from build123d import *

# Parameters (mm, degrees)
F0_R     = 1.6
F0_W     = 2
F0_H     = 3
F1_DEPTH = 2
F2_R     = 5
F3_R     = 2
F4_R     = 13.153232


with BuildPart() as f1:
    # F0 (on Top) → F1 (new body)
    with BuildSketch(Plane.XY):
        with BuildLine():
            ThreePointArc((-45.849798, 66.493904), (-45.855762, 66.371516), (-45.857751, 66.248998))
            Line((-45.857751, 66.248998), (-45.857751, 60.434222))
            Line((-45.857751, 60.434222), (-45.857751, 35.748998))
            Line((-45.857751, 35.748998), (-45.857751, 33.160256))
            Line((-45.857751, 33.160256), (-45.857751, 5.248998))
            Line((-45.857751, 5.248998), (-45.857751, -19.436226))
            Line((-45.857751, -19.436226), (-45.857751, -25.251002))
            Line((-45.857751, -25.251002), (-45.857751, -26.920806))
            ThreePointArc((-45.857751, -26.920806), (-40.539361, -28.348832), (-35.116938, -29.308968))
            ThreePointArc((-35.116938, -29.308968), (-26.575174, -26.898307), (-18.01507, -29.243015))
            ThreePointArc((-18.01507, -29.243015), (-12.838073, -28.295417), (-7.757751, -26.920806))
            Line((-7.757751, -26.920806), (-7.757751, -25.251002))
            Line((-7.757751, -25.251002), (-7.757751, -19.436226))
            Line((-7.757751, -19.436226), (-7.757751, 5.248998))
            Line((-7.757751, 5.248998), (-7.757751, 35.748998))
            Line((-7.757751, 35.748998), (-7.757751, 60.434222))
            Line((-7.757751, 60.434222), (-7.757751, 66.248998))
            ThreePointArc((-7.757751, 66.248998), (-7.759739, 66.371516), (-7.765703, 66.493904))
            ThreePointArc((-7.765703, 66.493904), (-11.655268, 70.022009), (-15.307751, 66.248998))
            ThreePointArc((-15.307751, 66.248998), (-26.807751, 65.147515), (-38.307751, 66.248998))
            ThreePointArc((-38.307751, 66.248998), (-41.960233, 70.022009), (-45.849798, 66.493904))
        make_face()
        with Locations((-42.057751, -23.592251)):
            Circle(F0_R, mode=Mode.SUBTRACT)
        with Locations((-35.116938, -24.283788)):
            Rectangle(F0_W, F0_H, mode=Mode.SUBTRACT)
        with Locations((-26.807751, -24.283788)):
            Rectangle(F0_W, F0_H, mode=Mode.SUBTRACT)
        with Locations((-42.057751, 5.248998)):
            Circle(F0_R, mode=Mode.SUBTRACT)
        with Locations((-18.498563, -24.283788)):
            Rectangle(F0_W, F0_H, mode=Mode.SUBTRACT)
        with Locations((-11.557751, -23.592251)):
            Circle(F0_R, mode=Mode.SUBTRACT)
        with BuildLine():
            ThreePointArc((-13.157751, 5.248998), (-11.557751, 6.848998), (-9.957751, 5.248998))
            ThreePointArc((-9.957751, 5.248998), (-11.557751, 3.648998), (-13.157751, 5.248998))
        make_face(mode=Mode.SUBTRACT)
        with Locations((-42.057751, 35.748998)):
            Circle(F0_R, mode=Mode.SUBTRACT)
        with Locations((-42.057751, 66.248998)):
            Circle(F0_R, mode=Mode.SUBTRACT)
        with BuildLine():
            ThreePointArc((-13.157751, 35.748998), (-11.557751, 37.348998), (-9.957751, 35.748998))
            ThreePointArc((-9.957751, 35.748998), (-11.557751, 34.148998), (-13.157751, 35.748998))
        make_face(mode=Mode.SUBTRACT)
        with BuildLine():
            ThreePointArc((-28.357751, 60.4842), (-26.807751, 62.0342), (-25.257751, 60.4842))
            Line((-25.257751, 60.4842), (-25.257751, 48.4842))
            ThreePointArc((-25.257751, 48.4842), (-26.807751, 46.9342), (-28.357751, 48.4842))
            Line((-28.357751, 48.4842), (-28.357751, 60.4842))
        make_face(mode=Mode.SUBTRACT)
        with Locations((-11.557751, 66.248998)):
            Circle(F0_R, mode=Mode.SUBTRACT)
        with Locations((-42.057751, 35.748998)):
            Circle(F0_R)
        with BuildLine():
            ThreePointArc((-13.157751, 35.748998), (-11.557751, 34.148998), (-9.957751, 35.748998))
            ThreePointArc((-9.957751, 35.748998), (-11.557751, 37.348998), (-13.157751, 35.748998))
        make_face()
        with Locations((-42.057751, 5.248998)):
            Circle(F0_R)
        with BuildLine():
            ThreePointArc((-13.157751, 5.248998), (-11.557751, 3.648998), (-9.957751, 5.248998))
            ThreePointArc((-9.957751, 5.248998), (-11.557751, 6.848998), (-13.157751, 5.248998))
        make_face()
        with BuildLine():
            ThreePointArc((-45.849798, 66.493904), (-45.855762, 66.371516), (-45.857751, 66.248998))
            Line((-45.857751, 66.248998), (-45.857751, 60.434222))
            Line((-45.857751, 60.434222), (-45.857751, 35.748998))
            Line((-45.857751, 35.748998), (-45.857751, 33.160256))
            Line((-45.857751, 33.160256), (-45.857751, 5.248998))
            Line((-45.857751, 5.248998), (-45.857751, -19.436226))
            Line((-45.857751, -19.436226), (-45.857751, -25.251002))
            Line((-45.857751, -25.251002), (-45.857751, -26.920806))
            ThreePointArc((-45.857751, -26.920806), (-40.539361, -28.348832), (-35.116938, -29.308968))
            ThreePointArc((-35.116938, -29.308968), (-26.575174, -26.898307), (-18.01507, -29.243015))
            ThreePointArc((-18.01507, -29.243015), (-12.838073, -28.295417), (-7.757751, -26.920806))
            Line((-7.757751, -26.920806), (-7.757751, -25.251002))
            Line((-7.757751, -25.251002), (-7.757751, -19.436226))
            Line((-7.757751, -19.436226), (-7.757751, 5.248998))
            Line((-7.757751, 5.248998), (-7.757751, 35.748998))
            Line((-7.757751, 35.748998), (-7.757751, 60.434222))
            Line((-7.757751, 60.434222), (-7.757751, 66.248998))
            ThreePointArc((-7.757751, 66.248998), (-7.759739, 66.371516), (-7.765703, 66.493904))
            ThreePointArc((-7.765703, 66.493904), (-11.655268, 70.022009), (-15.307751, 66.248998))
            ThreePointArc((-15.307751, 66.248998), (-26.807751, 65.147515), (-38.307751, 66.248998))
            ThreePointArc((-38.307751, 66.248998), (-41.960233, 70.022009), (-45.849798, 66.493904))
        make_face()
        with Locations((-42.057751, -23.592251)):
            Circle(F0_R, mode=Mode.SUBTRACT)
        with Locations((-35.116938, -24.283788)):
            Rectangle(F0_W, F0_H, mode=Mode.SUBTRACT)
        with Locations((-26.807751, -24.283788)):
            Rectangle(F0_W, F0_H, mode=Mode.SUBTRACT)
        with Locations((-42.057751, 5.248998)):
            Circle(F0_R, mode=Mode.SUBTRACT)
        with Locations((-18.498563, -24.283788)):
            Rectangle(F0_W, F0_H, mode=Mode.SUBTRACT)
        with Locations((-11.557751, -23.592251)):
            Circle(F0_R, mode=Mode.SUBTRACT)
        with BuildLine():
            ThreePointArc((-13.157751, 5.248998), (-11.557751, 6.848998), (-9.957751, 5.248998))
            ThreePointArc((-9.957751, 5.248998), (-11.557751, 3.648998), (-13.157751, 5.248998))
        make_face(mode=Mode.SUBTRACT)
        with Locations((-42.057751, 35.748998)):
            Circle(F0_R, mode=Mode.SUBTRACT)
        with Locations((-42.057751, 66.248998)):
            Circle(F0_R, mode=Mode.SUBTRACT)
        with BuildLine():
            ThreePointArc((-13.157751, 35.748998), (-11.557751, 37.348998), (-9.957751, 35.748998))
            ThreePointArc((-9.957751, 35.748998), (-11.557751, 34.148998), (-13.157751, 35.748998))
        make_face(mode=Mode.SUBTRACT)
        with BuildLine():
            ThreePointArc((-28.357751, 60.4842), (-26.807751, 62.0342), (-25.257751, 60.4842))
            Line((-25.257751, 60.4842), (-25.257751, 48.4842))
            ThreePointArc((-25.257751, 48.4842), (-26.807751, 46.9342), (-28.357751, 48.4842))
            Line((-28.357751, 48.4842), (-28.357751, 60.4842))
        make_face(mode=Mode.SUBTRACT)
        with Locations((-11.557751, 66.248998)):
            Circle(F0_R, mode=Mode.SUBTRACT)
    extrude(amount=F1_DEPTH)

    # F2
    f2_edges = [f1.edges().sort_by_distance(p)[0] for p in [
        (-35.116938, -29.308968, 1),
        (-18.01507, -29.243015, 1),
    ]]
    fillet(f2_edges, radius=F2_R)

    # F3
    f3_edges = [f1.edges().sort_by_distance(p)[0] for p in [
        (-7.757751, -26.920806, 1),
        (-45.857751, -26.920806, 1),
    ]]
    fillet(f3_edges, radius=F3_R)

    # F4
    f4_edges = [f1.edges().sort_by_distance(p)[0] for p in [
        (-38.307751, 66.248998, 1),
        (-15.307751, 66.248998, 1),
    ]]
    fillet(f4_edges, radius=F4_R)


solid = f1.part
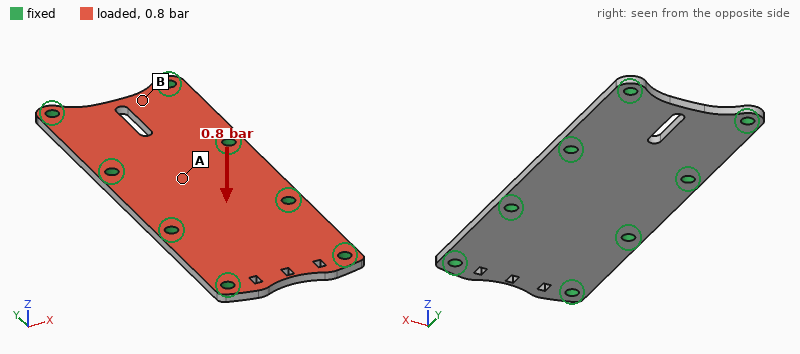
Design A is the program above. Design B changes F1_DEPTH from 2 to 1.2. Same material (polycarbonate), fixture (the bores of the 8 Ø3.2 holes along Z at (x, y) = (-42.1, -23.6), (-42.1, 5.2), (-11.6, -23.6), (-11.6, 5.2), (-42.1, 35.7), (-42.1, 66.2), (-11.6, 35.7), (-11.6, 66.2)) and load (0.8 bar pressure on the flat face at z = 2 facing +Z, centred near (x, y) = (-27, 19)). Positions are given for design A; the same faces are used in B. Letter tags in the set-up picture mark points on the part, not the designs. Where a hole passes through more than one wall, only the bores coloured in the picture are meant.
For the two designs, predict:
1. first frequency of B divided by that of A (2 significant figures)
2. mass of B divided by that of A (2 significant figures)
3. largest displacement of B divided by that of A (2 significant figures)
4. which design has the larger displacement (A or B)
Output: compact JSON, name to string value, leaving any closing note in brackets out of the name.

{"first frequency of B divided by that of A": "0.62", "mass of B divided by that of A": "0.60", "largest displacement of B divided by that of A": "4.3", "which design has the larger displacement": "B"}
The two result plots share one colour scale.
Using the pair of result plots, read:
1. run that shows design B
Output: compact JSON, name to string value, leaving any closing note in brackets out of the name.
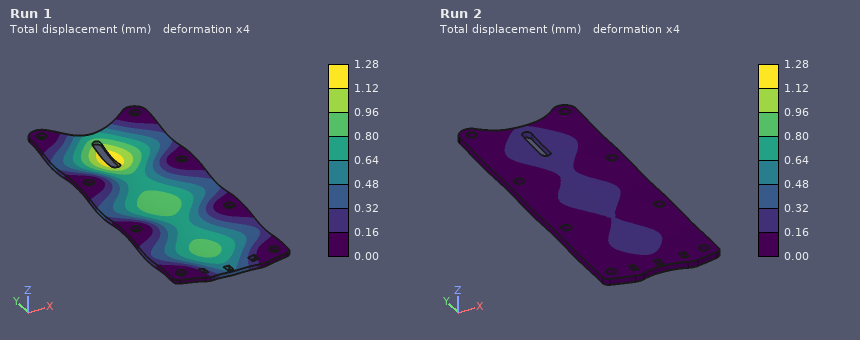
{"run that shows design B": "Run 1"}
